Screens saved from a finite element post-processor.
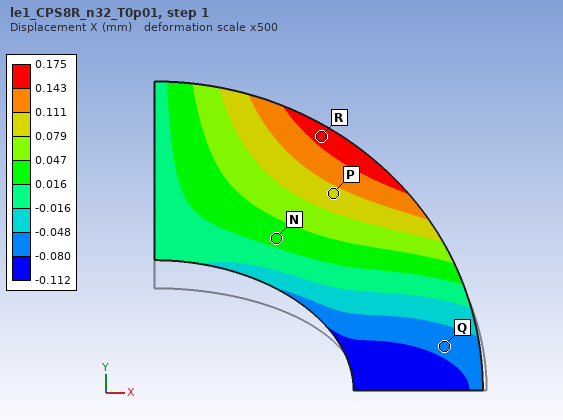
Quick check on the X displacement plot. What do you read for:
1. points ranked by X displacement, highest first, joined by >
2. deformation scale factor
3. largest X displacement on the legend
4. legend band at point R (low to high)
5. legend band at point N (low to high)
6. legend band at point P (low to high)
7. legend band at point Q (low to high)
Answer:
R > P > N > Q
500
0.175 mm
0.143 to 0.175 mm
0.016 to 0.047 mm
0.079 to 0.111 mm
-0.080 to -0.048 mm
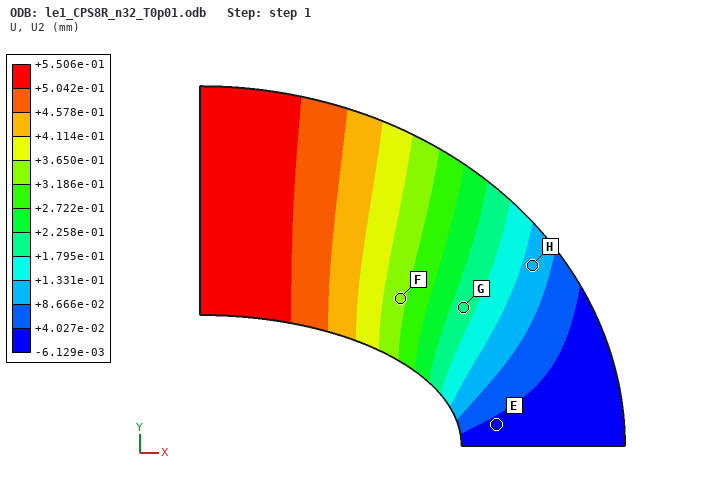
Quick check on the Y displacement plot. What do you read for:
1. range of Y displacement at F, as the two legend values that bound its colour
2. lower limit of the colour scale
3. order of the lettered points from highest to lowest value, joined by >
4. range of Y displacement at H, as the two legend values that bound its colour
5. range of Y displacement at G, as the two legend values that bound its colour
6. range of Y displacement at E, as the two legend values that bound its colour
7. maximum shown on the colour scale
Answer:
+3.186e-01 to +3.650e-01 mm
-6.129e-03 mm
F > G > H > E
+8.666e-02 to +1.331e-01 mm
+1.795e-01 to +2.258e-01 mm
-6.129e-03 to +4.027e-02 mm
+5.506e-01 mm
